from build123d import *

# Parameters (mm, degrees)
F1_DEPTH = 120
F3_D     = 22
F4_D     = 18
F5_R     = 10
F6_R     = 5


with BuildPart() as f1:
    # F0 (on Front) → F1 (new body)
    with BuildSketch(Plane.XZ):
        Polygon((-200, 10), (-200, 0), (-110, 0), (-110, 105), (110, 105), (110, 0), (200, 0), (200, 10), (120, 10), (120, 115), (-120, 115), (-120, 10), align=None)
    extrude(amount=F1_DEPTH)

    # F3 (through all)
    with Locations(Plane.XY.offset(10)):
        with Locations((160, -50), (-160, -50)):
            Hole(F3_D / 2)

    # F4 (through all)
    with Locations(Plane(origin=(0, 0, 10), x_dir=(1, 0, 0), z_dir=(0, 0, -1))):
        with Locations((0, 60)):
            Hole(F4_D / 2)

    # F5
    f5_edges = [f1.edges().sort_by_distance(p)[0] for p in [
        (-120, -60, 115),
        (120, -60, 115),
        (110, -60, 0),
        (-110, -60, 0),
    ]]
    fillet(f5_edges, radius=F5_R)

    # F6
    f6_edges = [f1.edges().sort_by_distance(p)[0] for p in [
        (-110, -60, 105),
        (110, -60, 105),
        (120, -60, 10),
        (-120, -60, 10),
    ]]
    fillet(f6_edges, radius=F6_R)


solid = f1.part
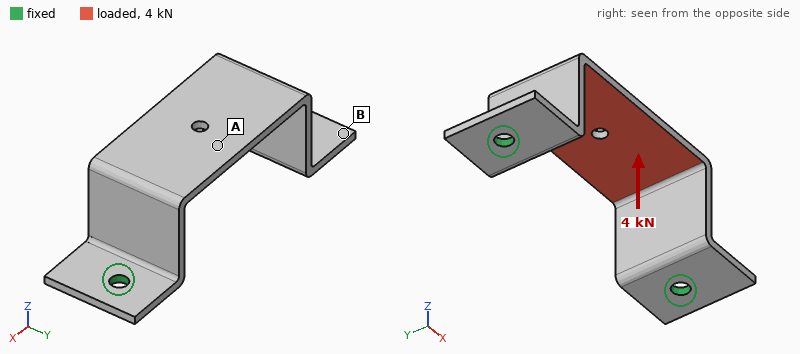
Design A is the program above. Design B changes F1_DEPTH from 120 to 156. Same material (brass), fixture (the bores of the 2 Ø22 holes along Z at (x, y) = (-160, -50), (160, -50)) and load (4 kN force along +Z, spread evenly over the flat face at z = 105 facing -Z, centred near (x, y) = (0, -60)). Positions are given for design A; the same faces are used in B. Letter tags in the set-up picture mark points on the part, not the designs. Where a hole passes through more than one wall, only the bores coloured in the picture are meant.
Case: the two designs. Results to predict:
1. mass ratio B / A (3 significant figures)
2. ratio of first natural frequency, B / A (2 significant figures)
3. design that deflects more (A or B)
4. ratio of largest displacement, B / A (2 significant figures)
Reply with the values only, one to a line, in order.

1.30
0.83
B
1.2
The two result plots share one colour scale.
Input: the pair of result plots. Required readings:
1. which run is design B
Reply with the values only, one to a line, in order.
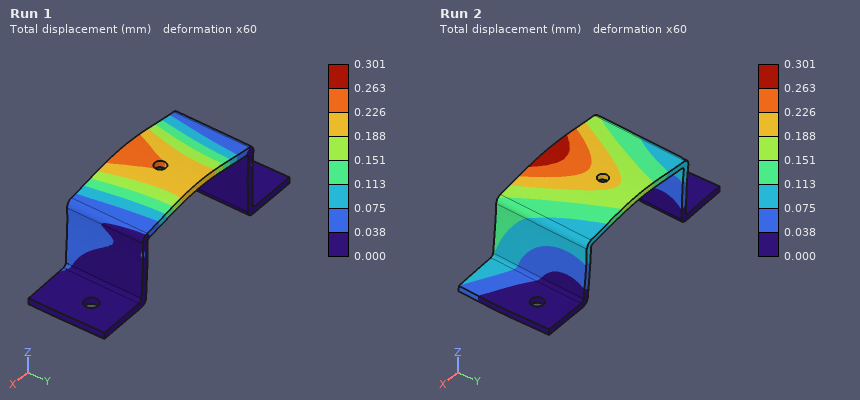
Run 2
